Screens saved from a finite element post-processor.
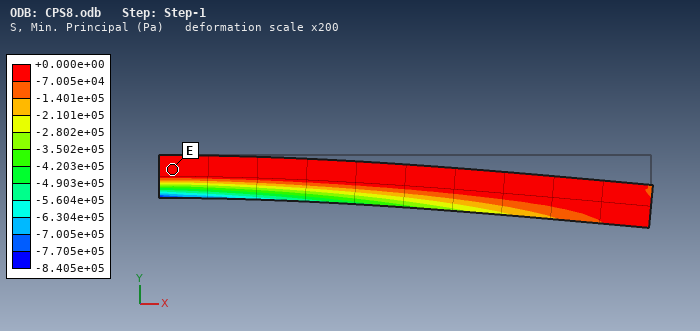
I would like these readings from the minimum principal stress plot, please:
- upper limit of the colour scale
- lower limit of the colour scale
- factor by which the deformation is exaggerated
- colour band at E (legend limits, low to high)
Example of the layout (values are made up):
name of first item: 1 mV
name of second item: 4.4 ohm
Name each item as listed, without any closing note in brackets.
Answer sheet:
upper limit of the colour scale: +0.000e+00 Pa
lower limit of the colour scale: -8.405e+05 Pa
factor by which the deformation is exaggerated: 200
colour band at E: -7.005e+04 to +0.000e+00 Pa
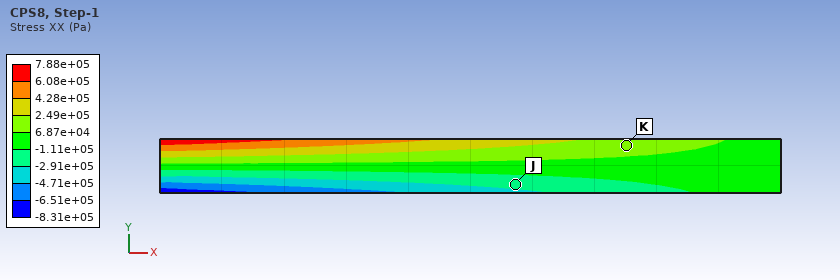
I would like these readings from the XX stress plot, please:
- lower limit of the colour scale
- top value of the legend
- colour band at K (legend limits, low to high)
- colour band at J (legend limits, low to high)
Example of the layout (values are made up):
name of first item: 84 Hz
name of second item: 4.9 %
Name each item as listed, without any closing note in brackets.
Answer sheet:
lower limit of the colour scale: -8.31e+05 Pa
top value of the legend: 7.88e+05 Pa
colour band at K: 6.87e+04 to 2.49e+05 Pa
colour band at J: -2.91e+05 to -1.11e+05 Pa
